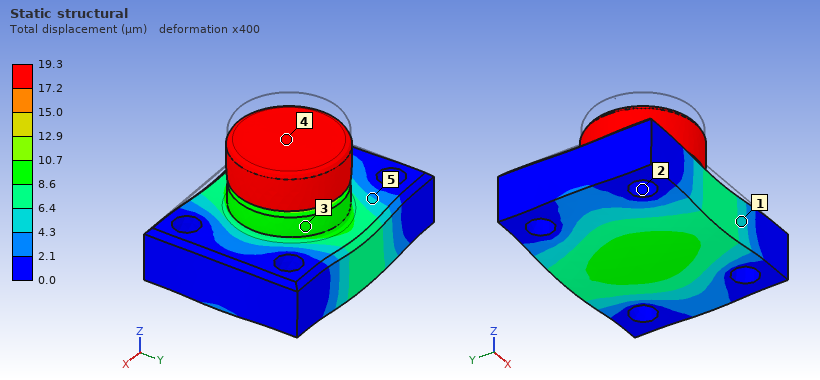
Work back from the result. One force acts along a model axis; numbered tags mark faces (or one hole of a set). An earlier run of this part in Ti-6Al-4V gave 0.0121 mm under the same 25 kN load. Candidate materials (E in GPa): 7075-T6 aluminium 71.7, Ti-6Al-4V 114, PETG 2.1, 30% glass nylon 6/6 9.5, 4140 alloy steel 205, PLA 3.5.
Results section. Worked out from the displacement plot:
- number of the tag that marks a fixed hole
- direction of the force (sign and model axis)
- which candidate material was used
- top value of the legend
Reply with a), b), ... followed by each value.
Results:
a) 2
b) -Z
c) 7075-T6 aluminium
d) 19.3 µm
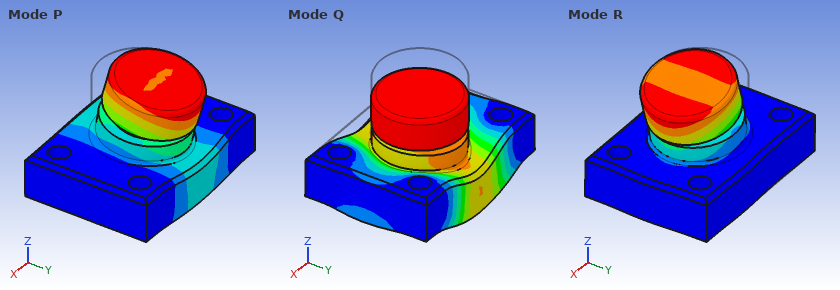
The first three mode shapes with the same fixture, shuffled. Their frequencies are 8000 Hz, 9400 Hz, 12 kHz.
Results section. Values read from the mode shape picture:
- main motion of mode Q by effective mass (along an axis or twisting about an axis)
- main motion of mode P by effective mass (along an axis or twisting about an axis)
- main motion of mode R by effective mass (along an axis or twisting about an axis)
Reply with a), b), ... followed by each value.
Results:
a) along Z
b) along Y
c) along X
